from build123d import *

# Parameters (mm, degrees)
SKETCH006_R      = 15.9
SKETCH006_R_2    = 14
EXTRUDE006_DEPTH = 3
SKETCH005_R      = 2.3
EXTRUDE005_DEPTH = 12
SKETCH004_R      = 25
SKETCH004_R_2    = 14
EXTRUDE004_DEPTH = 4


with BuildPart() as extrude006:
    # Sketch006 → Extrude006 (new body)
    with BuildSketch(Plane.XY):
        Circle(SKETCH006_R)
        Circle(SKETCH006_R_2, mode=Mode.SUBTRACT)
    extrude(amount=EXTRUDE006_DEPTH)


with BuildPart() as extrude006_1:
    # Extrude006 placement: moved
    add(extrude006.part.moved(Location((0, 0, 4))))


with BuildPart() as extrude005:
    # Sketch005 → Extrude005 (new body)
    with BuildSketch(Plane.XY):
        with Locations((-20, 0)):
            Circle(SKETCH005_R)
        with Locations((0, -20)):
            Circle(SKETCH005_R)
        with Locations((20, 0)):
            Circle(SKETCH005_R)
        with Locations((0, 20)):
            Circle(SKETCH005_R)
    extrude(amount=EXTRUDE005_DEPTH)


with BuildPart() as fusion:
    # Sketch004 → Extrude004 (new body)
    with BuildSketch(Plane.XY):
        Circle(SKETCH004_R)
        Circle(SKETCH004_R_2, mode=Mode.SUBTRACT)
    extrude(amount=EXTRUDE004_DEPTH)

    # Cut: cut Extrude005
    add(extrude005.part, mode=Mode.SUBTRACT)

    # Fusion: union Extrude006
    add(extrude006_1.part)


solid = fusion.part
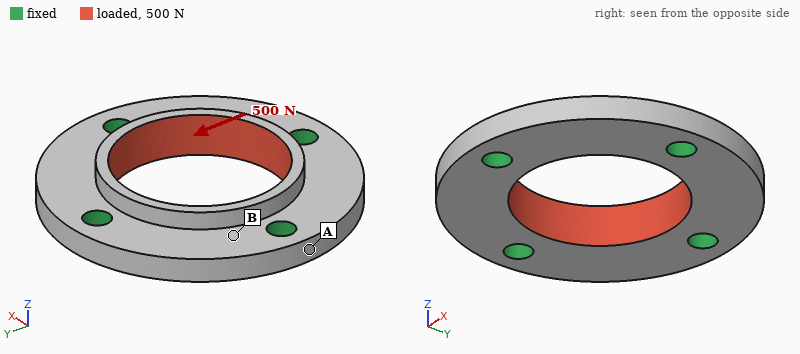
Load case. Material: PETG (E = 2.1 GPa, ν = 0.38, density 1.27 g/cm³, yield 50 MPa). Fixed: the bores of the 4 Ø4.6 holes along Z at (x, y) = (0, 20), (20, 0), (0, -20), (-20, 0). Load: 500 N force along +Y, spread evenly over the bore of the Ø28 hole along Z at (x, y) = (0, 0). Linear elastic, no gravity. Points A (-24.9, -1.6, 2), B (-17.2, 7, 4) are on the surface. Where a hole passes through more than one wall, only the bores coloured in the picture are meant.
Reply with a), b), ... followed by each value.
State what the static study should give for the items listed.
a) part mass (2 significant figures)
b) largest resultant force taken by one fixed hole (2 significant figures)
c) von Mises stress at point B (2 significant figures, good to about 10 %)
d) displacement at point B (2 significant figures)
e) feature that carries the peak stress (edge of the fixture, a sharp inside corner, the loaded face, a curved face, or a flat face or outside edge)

a) 7.2 g
b) 140 N
c) 1.9 MPa
d) 11 µm
e) edge of the fixture
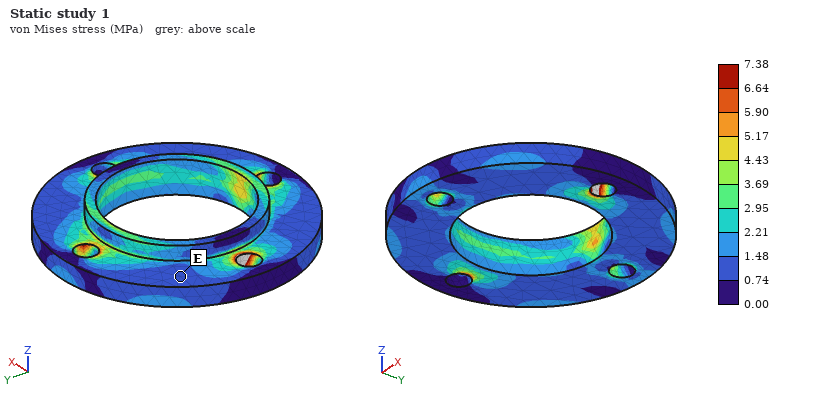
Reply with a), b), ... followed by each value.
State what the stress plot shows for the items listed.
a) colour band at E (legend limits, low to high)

a) 0.74 to 1.48 MPa
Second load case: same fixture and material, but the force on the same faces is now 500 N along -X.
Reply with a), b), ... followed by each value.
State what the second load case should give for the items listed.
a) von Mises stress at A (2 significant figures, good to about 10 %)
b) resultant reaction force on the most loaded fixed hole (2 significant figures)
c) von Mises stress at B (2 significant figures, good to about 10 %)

a) 1.5 MPa
b) 140 N
c) 2.5 MPa
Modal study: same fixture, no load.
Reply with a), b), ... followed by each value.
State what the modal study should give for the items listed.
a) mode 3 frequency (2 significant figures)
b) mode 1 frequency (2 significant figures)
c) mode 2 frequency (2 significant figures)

a) 5400 Hz
b) 5100 Hz
c) 5300 Hz
